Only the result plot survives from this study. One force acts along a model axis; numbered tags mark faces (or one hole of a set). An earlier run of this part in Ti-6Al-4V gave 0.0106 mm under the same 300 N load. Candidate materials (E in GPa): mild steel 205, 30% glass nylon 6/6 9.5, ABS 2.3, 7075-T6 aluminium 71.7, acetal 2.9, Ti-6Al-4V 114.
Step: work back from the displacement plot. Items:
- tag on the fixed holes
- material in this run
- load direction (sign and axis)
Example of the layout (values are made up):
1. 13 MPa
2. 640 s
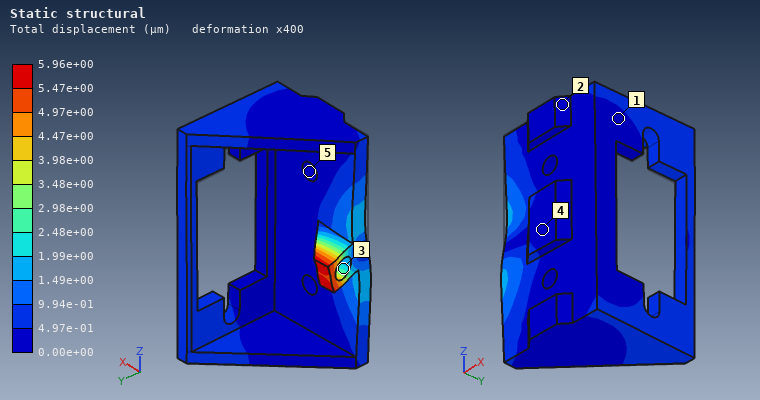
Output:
1. 5
2. mild steel
3. -Z
